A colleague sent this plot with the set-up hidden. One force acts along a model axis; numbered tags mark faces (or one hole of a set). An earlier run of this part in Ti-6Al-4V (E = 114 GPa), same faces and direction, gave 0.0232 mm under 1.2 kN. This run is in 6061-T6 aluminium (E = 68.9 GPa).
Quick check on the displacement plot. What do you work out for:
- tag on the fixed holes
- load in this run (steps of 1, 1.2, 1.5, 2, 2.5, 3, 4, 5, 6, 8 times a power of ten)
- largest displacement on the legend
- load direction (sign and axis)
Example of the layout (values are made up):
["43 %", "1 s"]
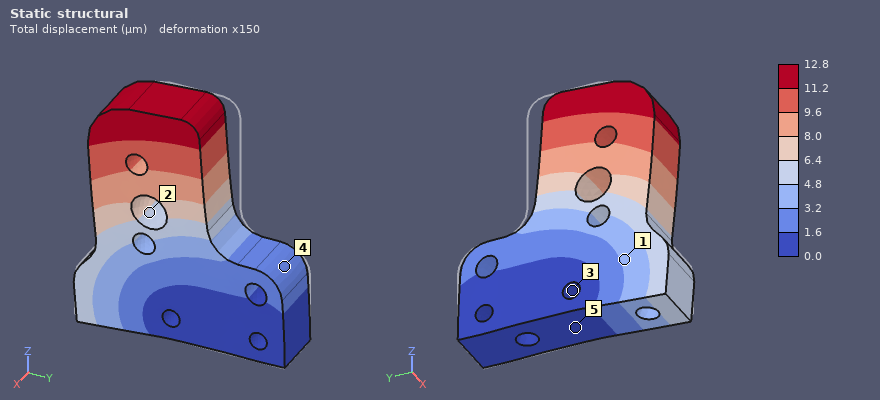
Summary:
["3", "400 N", "12.8 µm", "-Y"]
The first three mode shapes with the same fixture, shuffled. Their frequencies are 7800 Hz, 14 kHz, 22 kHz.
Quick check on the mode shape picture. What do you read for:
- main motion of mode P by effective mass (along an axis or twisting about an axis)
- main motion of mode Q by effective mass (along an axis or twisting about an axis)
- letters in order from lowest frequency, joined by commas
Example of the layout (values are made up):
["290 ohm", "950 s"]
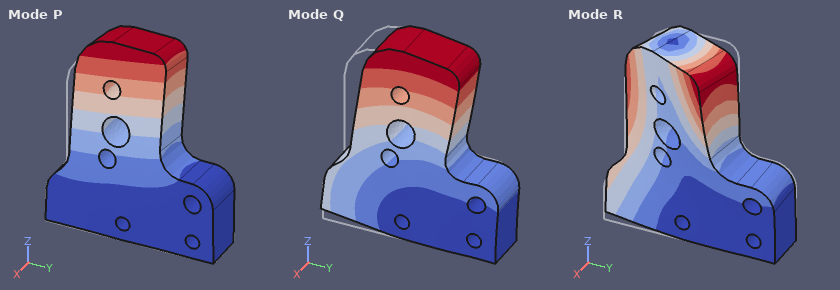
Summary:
["along X", "along Y", "P, Q, R"]
